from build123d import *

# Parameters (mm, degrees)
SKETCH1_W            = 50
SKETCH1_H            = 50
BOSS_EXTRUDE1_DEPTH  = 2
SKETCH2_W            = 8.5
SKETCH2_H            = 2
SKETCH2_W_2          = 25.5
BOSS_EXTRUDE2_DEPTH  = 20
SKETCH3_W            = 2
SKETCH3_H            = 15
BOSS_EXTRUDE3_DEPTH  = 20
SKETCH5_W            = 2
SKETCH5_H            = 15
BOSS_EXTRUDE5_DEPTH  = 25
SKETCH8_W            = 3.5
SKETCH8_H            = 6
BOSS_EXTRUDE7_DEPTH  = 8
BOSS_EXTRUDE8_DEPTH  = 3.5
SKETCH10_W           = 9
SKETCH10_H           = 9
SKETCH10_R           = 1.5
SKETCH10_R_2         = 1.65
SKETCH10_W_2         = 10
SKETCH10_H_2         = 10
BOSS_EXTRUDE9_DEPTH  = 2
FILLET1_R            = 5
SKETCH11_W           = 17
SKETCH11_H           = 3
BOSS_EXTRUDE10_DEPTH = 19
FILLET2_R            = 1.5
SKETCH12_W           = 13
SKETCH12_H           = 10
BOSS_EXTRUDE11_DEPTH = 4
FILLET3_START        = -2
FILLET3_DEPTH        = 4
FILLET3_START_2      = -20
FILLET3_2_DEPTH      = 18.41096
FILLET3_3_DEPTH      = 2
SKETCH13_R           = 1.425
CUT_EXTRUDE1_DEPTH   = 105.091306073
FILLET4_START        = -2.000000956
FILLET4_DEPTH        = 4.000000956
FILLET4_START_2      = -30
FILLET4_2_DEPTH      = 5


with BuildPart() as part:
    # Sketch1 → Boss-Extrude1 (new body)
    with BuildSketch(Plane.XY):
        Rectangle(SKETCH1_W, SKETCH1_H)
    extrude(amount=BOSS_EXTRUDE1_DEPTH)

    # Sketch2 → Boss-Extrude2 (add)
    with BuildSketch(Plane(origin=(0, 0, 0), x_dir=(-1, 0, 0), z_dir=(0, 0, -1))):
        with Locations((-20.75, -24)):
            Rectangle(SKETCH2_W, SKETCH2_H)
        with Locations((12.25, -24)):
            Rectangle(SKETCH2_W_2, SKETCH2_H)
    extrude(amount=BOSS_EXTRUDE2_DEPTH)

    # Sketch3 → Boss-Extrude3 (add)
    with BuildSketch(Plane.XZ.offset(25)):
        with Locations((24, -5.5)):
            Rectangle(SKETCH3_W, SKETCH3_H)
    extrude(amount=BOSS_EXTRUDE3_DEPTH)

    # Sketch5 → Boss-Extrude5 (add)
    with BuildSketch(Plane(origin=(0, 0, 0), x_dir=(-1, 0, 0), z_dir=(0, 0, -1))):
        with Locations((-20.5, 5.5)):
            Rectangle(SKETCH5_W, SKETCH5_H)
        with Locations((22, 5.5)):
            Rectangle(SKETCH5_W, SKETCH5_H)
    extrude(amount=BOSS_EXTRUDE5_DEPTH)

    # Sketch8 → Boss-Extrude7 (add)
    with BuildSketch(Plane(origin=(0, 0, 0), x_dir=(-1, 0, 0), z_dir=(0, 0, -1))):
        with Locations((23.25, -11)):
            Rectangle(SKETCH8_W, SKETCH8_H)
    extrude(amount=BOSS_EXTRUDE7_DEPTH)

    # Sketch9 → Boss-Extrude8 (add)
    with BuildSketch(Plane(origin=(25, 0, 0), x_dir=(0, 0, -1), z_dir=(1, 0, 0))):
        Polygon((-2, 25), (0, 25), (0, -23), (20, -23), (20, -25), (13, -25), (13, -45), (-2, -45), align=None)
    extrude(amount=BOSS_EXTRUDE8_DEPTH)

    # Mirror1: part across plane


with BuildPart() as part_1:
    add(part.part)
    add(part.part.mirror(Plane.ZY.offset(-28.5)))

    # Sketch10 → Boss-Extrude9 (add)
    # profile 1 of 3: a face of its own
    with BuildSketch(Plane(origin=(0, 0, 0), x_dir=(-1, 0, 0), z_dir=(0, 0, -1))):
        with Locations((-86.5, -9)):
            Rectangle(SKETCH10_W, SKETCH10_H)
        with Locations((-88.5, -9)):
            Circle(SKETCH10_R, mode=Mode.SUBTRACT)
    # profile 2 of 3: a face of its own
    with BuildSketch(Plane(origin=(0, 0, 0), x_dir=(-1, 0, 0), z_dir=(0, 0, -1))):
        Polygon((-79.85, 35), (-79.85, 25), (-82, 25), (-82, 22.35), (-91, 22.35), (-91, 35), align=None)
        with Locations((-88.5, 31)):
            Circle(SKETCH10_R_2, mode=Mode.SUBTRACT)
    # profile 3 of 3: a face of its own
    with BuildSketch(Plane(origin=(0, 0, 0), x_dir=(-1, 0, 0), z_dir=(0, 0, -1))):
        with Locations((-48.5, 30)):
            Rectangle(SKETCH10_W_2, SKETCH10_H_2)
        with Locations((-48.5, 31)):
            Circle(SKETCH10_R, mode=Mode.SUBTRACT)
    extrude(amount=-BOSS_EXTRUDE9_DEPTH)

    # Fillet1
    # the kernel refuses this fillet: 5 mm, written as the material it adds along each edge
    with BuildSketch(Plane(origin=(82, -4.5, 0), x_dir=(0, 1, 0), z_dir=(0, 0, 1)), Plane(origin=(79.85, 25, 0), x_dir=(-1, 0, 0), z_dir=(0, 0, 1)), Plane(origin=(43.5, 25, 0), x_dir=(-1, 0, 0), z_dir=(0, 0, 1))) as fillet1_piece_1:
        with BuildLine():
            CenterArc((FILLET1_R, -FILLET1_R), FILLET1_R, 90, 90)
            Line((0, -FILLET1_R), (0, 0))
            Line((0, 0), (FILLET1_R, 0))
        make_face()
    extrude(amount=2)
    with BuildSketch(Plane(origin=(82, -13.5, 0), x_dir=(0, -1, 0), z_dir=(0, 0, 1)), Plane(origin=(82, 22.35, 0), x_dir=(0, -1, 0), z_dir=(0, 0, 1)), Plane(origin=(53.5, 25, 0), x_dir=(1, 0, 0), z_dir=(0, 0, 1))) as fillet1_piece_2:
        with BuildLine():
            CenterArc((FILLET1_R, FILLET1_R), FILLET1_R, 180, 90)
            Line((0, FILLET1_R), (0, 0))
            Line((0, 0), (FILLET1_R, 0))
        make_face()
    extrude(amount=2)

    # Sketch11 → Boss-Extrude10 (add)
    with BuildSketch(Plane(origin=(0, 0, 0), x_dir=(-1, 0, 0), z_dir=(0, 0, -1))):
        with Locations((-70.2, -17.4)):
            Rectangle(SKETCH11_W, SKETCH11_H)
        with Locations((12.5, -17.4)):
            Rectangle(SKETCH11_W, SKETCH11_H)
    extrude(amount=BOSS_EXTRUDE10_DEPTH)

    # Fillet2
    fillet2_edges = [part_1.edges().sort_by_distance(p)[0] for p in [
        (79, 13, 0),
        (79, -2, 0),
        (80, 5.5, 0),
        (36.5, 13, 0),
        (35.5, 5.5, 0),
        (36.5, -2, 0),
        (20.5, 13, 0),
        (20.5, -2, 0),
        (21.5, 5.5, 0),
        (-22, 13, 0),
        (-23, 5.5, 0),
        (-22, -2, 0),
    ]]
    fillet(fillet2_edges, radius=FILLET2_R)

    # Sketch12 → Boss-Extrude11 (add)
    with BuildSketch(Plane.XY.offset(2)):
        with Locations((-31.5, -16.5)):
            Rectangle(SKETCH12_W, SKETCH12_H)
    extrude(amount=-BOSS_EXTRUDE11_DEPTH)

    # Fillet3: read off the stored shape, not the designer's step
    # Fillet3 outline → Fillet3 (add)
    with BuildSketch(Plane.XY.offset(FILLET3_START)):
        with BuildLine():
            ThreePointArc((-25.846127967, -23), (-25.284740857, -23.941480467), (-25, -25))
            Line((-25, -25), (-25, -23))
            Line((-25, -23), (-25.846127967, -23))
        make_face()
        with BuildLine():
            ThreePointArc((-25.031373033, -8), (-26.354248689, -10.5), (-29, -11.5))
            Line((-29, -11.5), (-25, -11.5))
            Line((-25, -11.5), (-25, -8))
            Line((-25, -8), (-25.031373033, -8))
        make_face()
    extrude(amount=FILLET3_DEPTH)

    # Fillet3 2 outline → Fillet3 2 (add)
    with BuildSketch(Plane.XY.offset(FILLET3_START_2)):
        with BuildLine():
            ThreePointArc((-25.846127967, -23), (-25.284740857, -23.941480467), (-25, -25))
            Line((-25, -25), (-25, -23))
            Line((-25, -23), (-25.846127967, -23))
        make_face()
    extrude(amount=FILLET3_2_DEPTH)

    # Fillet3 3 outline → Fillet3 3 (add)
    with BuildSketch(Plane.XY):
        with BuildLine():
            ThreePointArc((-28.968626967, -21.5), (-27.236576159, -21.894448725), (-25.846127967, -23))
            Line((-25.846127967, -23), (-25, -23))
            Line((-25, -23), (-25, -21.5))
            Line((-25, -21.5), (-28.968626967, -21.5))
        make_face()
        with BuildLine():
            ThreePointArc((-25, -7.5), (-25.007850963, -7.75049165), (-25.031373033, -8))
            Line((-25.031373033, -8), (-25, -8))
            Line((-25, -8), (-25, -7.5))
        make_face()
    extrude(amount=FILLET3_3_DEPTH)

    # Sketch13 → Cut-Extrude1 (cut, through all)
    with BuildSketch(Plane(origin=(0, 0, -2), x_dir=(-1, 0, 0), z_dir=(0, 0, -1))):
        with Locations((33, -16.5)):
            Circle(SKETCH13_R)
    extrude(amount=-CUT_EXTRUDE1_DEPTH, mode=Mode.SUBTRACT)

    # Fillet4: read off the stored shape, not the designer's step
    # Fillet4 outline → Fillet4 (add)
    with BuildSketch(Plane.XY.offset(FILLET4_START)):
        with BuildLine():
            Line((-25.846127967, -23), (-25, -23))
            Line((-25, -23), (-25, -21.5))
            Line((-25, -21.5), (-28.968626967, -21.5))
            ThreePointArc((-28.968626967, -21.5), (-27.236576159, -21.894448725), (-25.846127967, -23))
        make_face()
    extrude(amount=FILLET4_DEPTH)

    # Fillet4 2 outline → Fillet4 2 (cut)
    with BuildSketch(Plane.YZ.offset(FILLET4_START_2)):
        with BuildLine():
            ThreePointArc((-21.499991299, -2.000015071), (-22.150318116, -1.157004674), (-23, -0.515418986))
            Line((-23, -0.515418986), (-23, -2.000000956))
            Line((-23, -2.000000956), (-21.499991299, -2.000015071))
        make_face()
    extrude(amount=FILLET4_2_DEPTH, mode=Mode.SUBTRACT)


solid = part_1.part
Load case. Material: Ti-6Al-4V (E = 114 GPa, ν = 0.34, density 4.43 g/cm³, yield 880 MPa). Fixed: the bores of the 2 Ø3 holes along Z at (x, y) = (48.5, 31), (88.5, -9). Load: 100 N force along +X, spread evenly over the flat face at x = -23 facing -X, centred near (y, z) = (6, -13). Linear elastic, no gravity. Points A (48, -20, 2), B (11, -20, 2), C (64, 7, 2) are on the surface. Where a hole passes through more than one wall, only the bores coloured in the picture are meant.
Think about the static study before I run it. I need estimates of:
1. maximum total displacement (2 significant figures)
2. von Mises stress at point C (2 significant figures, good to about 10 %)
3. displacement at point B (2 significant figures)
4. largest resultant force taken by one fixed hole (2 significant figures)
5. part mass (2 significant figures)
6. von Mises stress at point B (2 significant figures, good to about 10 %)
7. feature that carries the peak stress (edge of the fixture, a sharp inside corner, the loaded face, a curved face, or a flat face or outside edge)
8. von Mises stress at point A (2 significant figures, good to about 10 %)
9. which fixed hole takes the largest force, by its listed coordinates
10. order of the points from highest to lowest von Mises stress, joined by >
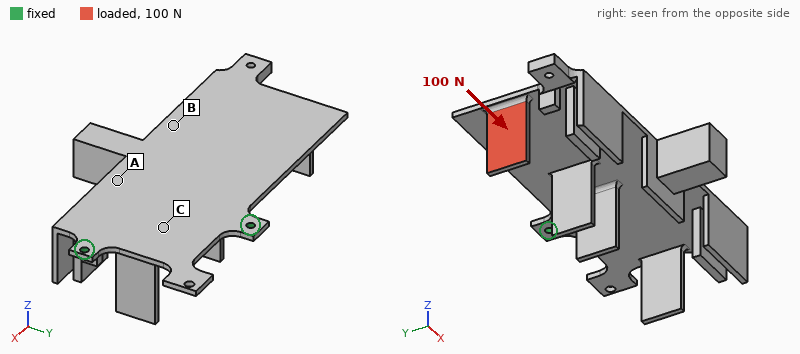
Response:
1.7 mm
11 MPa
0.58 mm
63 N
100 g
52 MPa
the loaded face
39 MPa
(88.5, -9)
B > A > C
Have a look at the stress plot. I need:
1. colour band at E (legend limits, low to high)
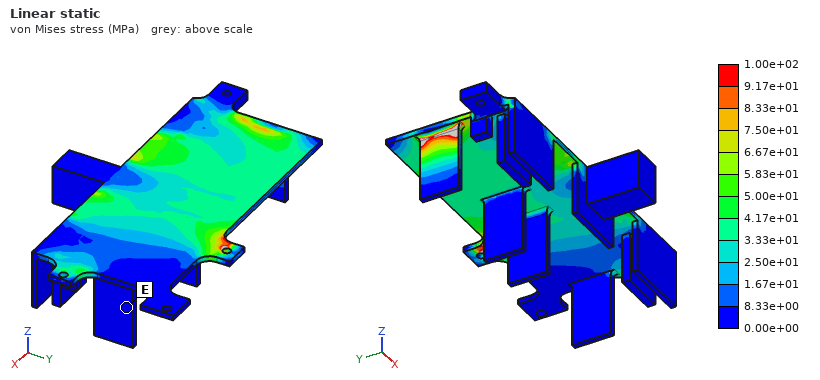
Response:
0.00e+00 to 8.33e+00 MPa
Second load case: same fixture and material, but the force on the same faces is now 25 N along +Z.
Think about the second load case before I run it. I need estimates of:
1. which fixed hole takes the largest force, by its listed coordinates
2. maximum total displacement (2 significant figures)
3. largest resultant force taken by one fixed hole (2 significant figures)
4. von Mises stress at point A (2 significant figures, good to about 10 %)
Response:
(48.5, 31)
1.8 mm
40 N
42 MPa
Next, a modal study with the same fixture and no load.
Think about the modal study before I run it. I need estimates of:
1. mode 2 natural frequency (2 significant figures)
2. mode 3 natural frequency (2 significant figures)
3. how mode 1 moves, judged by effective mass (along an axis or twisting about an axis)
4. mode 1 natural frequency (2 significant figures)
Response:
340 Hz
700 Hz
along Z
110 Hz
